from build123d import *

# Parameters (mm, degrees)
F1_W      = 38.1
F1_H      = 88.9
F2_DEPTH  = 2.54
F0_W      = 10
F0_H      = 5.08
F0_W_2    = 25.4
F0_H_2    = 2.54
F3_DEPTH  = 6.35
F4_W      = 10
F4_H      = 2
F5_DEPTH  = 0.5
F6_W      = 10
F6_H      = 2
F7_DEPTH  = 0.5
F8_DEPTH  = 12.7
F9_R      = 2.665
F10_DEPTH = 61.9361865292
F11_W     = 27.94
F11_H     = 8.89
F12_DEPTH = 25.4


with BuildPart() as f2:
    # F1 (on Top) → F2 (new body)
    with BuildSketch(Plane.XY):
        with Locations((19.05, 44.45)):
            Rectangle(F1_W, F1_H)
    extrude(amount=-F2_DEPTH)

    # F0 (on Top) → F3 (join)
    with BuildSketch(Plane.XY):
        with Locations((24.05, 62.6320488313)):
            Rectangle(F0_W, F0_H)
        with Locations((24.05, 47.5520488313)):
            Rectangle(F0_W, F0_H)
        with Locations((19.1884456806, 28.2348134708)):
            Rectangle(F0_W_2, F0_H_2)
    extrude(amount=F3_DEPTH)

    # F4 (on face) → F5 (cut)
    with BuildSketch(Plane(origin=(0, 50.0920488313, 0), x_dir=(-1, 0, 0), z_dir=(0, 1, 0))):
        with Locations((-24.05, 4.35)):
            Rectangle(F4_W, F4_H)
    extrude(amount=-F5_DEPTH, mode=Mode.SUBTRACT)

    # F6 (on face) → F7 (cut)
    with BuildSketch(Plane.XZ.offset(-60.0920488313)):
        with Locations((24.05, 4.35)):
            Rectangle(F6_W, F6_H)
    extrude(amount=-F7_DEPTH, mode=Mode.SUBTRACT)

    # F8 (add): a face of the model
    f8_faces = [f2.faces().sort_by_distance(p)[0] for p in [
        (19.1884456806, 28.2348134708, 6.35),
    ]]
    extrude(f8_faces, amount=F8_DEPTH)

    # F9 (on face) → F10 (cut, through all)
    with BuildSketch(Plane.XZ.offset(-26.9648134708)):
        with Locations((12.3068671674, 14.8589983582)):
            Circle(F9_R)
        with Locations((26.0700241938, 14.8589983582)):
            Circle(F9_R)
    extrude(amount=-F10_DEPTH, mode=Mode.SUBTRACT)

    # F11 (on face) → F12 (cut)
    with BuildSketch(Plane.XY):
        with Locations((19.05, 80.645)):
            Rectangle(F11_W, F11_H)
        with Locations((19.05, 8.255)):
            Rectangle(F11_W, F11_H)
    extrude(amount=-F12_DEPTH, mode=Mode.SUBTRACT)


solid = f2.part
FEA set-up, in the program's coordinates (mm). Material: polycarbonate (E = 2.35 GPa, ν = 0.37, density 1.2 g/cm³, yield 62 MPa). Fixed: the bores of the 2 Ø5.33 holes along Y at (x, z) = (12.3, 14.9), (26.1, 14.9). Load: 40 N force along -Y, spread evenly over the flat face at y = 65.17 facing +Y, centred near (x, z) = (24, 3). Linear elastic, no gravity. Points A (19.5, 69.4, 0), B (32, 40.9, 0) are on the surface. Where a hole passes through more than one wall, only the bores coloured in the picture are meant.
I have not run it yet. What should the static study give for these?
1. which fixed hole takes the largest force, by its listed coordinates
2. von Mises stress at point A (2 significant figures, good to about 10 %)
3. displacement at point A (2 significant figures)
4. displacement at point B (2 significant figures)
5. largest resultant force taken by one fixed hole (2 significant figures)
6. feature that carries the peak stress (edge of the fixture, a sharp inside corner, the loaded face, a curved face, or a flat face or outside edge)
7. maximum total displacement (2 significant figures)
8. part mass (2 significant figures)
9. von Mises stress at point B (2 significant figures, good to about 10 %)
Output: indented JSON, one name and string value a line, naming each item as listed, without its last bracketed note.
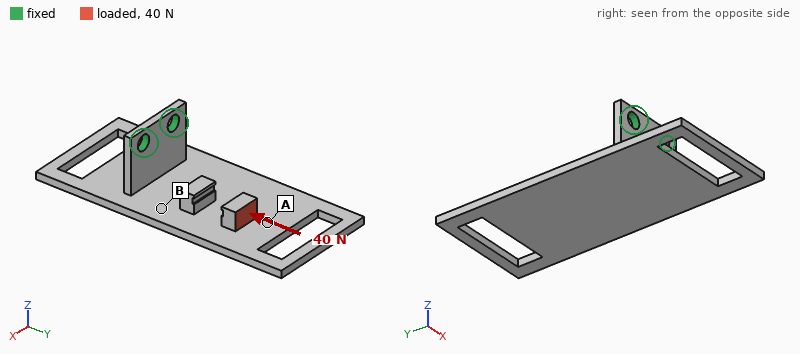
{
  "which fixed hole takes the largest force, by its listed coordinates": "(26.1, 14.9)",
  "von Mises stress at point A": "1.3 MPa",
  "displacement at point A": "0.54 mm",
  "displacement at point B": "0.41 mm",
  "largest resultant force taken by one fixed hole": "31 N",
  "feature that carries the peak stress": "a flat face or outside edge",
  "maximum total displacement": "1.0 mm",
  "part mass": "11 g",
  "von Mises stress at point B": "5.0 MPa"
}
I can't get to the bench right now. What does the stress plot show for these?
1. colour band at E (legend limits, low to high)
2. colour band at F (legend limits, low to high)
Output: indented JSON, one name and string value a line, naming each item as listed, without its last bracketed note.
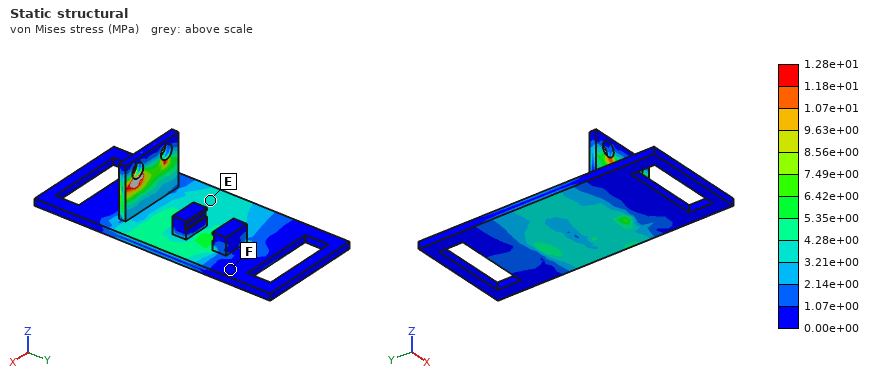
{
  "colour band at E": "3.21e+00 to 4.28e+00 MPa",
  "colour band at F": "0.00e+00 to 1.07e+00 MPa"
}
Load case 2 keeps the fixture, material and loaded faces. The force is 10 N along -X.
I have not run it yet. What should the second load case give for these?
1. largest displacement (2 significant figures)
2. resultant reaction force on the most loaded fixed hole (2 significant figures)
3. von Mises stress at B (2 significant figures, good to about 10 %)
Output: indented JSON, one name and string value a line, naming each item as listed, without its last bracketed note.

{
  "largest displacement": "1.1 mm",
  "resultant reaction force on the most loaded fixed hole": "23 N",
  "von Mises stress at B": "1.7 MPa"
}
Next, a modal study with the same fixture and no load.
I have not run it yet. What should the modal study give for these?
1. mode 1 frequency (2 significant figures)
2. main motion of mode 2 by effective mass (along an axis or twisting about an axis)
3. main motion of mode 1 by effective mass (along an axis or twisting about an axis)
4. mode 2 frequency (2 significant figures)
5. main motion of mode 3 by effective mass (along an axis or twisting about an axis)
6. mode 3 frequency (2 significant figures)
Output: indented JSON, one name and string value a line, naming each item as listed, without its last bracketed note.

{
  "mode 1 frequency": "120 Hz",
  "main motion of mode 2 by effective mass": "along X",
  "main motion of mode 1 by effective mass": "along Z",
  "mode 2 frequency": "250 Hz",
  "main motion of mode 3 by effective mass": "along Y",
  "mode 3 frequency": "480 Hz"
}
